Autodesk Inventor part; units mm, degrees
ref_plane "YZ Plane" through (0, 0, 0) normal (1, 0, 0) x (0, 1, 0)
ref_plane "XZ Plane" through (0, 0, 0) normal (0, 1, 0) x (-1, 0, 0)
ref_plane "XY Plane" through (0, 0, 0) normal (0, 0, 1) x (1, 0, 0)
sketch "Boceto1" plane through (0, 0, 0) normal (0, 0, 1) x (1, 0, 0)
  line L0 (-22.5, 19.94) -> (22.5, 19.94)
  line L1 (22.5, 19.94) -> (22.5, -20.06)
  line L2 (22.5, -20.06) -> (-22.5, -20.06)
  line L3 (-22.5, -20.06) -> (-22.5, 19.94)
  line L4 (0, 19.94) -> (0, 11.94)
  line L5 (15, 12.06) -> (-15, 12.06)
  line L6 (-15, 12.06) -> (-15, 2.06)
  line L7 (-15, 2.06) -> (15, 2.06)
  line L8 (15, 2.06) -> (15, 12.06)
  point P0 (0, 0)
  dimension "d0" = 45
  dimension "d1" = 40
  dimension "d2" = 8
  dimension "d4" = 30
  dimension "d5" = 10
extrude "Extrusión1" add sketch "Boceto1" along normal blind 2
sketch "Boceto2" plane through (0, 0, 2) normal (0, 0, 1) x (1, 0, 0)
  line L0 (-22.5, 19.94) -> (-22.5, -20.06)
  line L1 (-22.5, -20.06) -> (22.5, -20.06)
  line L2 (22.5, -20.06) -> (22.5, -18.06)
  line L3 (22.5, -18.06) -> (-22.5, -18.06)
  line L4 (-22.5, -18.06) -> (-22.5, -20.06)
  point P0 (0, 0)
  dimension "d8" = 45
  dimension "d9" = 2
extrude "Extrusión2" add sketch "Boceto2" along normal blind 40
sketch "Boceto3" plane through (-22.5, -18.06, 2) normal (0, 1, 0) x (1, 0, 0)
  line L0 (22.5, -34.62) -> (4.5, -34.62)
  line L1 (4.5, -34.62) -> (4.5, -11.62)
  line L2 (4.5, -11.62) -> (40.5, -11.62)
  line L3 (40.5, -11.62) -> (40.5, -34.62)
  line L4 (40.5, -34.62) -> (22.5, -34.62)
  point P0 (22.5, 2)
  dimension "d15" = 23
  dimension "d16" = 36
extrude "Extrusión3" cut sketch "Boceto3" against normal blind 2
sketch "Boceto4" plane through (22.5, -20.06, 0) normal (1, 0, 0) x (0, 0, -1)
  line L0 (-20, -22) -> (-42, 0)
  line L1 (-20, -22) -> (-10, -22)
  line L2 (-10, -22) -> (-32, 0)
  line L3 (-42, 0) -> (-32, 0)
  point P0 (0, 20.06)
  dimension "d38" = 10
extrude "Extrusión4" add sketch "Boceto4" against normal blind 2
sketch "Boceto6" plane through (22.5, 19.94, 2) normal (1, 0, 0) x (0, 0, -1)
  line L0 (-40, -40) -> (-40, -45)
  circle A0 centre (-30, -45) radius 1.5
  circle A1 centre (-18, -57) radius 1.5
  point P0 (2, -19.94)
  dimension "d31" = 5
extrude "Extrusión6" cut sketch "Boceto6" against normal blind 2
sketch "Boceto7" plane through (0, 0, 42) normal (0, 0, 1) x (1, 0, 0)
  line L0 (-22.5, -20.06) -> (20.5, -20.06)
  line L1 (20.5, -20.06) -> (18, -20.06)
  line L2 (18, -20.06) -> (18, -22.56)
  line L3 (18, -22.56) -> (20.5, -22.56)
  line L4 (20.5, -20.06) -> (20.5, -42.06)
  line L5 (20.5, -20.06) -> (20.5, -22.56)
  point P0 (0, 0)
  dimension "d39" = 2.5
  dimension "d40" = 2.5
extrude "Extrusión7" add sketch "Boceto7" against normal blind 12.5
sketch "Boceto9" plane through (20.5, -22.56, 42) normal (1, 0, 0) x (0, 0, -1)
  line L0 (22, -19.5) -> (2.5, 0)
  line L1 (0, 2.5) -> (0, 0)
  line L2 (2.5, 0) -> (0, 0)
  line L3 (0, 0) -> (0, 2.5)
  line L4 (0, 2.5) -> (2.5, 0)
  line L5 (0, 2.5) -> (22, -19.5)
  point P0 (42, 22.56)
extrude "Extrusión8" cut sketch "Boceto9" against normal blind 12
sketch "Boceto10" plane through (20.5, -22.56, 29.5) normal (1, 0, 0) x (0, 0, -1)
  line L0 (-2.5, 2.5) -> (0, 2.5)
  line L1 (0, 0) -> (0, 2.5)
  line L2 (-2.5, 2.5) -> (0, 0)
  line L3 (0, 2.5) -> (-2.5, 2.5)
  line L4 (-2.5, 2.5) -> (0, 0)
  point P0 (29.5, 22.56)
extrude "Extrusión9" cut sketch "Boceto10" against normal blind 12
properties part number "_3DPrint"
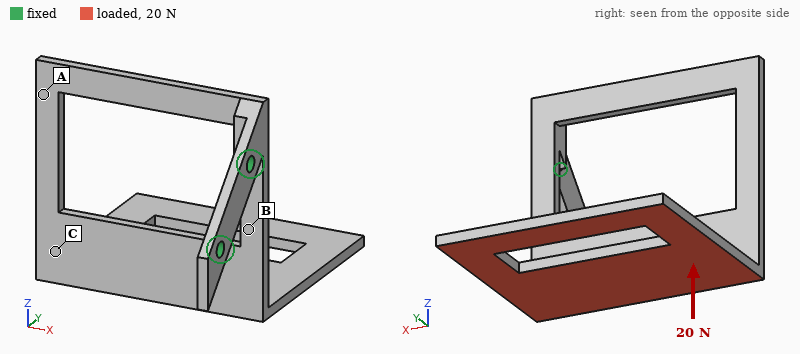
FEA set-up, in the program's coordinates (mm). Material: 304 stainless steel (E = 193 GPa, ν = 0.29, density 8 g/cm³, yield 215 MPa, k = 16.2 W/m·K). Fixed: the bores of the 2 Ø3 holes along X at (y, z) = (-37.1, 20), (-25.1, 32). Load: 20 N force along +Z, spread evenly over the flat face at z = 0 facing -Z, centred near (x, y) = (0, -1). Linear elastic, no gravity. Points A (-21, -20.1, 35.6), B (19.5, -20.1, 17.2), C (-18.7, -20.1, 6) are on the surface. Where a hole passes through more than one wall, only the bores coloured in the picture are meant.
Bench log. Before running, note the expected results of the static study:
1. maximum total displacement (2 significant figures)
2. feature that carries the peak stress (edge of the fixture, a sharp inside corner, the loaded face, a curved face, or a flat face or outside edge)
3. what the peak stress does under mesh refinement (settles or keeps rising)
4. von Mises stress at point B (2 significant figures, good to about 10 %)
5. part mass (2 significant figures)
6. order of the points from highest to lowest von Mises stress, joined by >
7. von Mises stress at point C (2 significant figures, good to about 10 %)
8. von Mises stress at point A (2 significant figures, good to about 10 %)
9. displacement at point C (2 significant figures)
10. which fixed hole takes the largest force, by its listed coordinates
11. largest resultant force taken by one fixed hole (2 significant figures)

0.55 mm
edge of the fixture
keeps rising
73 MPa
43 g
B > A > C
15 MPa
36 MPa
0.22 mm
(-25.1, 32)
25 N
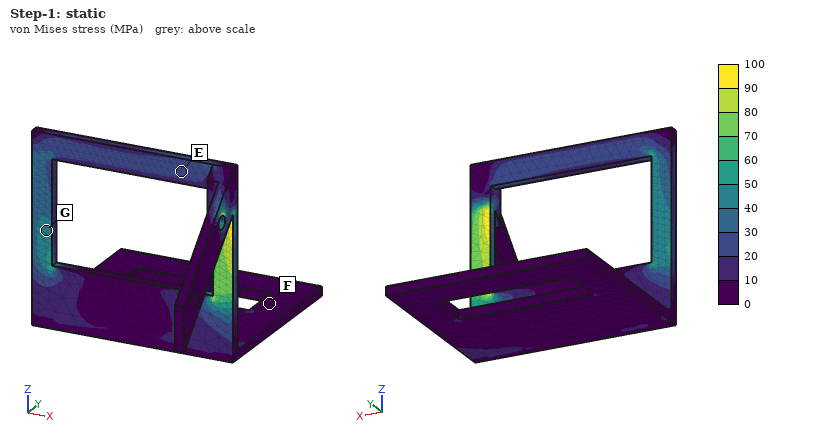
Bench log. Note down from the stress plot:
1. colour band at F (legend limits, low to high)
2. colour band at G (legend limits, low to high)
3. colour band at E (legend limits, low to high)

0 to 10 MPa
40 to 50 MPa
20 to 30 MPa
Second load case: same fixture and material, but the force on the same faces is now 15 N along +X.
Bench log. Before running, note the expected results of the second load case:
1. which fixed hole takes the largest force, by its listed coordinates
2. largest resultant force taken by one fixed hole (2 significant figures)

(-25.1, 32)
16 N
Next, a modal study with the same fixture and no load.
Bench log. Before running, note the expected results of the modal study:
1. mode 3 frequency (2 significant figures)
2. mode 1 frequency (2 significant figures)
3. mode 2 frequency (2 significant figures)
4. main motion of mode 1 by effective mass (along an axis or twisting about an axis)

520 Hz
150 Hz
270 Hz
along Y
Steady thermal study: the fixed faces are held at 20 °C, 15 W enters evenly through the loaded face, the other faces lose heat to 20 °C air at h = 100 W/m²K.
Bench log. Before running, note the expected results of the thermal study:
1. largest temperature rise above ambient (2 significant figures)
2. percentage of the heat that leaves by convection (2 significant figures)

67 K
100 %
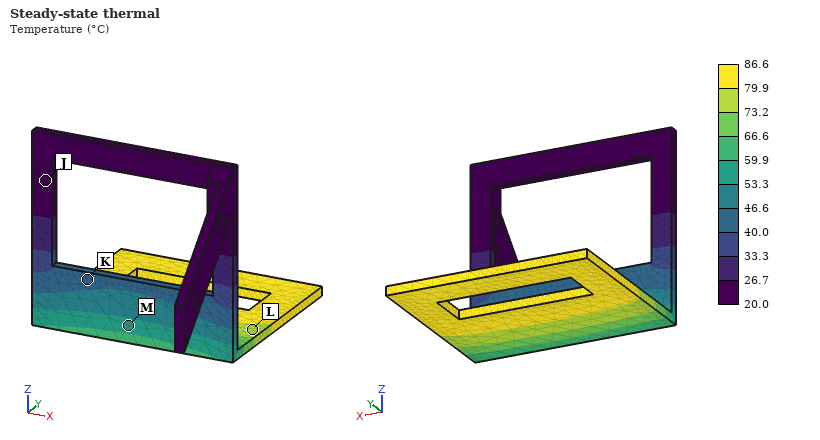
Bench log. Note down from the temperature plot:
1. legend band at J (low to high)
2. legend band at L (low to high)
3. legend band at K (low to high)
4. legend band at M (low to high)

20.0 to 26.7 °C
73.2 to 79.9 °C
40.0 to 46.6 °C
53.3 to 59.9 °C
